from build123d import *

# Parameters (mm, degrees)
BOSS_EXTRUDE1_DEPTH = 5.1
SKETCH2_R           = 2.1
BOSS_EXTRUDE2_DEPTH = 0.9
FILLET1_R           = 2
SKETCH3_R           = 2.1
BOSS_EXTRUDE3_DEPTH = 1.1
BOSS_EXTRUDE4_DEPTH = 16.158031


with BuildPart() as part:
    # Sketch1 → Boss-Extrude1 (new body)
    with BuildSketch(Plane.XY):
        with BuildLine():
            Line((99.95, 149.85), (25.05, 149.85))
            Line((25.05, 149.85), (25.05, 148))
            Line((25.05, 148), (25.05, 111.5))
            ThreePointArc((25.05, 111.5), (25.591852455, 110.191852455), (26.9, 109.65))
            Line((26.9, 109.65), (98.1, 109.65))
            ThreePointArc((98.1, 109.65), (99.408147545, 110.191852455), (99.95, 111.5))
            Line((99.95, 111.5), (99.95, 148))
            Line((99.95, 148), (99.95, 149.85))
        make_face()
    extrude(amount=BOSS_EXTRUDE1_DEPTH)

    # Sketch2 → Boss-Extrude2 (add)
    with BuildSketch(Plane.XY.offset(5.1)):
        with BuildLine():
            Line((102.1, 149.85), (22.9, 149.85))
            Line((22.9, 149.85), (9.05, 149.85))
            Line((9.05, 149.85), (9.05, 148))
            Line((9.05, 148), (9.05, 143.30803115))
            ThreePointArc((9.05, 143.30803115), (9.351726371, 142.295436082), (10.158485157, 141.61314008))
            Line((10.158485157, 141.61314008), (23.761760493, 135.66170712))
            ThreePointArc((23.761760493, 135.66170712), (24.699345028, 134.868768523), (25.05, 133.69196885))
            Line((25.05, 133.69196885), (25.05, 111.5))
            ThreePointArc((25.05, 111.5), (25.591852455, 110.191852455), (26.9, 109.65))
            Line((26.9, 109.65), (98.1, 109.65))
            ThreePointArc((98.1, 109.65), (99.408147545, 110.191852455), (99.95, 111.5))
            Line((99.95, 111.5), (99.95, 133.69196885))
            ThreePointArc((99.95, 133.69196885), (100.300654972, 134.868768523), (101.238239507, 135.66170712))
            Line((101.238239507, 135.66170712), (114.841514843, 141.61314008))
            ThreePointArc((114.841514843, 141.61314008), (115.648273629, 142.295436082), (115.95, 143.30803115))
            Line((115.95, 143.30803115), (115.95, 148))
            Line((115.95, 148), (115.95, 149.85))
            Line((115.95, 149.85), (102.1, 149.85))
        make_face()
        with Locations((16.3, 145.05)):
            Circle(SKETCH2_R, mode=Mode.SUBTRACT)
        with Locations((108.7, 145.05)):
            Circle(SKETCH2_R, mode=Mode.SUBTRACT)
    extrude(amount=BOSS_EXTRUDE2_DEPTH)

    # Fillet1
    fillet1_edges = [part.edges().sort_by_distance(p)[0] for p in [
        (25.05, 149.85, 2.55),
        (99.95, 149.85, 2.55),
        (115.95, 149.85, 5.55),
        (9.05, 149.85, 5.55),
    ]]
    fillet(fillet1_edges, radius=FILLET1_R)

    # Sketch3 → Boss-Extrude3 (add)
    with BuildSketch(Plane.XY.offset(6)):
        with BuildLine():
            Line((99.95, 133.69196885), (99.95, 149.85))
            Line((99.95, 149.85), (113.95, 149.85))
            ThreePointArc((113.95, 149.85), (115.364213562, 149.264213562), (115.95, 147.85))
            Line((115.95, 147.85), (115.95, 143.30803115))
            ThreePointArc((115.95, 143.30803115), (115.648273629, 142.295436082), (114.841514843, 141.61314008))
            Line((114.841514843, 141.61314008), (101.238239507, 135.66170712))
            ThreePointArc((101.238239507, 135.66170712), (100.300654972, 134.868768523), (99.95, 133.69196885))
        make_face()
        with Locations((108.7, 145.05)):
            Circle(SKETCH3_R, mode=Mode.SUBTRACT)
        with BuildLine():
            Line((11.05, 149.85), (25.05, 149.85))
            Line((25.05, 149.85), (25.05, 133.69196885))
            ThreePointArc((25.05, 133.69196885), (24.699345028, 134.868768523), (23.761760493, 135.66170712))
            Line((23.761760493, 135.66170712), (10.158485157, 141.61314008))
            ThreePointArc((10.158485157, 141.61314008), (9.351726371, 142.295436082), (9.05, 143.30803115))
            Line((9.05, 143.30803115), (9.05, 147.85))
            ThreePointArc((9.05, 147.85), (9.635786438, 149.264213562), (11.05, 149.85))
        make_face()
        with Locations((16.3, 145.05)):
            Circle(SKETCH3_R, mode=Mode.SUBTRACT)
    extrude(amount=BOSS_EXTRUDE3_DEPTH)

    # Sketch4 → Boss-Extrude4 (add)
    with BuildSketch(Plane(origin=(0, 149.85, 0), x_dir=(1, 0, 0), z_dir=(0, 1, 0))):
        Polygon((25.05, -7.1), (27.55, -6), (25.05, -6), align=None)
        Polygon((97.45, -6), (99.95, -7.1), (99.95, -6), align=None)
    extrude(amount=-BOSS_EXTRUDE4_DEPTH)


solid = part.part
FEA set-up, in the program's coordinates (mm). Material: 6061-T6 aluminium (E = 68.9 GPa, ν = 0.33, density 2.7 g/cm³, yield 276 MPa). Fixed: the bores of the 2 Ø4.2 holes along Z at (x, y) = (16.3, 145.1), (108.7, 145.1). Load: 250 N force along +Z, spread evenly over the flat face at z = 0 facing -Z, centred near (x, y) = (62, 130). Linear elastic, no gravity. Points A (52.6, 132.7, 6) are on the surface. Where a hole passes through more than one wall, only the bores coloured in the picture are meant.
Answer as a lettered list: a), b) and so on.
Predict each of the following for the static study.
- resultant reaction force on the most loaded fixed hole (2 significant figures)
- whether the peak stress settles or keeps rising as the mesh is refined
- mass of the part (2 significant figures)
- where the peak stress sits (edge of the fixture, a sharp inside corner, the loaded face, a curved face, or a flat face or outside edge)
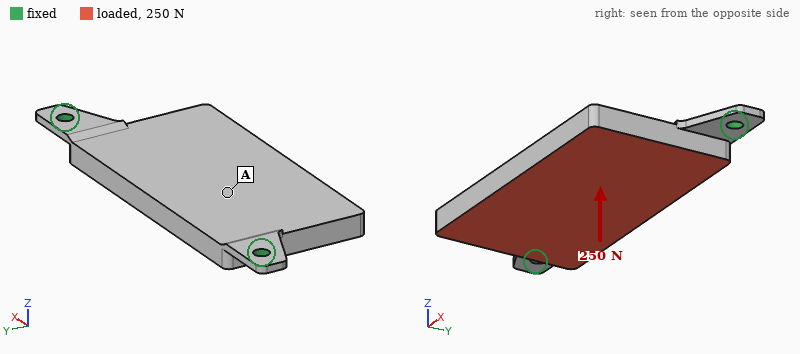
a) 270 N
b) keeps rising
c) 51 g
d) edge of the fixture
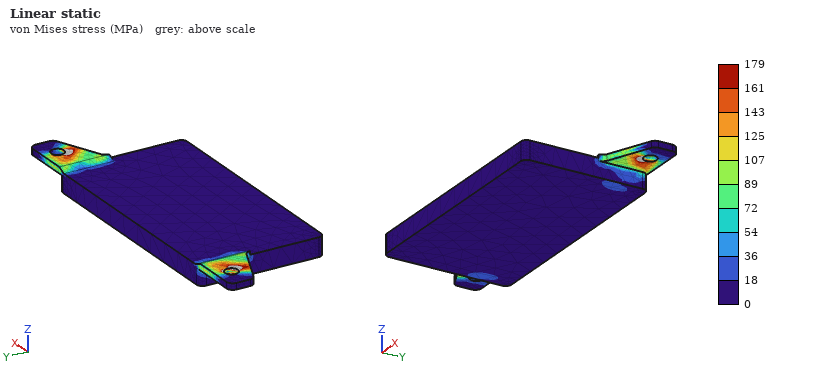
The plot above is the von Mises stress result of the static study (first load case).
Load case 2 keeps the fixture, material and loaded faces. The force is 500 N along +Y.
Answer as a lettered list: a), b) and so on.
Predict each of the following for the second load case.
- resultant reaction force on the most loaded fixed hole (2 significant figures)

a) 280 N
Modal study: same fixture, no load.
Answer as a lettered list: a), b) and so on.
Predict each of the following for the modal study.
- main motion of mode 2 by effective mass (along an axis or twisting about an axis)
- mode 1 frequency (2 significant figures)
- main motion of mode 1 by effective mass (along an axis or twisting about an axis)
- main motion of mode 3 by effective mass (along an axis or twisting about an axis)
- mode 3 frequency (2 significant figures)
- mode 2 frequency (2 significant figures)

a) along Z
b) 600 Hz
c) along Z
d) twisting about Y
e) 3200 Hz
f) 3000 Hz
